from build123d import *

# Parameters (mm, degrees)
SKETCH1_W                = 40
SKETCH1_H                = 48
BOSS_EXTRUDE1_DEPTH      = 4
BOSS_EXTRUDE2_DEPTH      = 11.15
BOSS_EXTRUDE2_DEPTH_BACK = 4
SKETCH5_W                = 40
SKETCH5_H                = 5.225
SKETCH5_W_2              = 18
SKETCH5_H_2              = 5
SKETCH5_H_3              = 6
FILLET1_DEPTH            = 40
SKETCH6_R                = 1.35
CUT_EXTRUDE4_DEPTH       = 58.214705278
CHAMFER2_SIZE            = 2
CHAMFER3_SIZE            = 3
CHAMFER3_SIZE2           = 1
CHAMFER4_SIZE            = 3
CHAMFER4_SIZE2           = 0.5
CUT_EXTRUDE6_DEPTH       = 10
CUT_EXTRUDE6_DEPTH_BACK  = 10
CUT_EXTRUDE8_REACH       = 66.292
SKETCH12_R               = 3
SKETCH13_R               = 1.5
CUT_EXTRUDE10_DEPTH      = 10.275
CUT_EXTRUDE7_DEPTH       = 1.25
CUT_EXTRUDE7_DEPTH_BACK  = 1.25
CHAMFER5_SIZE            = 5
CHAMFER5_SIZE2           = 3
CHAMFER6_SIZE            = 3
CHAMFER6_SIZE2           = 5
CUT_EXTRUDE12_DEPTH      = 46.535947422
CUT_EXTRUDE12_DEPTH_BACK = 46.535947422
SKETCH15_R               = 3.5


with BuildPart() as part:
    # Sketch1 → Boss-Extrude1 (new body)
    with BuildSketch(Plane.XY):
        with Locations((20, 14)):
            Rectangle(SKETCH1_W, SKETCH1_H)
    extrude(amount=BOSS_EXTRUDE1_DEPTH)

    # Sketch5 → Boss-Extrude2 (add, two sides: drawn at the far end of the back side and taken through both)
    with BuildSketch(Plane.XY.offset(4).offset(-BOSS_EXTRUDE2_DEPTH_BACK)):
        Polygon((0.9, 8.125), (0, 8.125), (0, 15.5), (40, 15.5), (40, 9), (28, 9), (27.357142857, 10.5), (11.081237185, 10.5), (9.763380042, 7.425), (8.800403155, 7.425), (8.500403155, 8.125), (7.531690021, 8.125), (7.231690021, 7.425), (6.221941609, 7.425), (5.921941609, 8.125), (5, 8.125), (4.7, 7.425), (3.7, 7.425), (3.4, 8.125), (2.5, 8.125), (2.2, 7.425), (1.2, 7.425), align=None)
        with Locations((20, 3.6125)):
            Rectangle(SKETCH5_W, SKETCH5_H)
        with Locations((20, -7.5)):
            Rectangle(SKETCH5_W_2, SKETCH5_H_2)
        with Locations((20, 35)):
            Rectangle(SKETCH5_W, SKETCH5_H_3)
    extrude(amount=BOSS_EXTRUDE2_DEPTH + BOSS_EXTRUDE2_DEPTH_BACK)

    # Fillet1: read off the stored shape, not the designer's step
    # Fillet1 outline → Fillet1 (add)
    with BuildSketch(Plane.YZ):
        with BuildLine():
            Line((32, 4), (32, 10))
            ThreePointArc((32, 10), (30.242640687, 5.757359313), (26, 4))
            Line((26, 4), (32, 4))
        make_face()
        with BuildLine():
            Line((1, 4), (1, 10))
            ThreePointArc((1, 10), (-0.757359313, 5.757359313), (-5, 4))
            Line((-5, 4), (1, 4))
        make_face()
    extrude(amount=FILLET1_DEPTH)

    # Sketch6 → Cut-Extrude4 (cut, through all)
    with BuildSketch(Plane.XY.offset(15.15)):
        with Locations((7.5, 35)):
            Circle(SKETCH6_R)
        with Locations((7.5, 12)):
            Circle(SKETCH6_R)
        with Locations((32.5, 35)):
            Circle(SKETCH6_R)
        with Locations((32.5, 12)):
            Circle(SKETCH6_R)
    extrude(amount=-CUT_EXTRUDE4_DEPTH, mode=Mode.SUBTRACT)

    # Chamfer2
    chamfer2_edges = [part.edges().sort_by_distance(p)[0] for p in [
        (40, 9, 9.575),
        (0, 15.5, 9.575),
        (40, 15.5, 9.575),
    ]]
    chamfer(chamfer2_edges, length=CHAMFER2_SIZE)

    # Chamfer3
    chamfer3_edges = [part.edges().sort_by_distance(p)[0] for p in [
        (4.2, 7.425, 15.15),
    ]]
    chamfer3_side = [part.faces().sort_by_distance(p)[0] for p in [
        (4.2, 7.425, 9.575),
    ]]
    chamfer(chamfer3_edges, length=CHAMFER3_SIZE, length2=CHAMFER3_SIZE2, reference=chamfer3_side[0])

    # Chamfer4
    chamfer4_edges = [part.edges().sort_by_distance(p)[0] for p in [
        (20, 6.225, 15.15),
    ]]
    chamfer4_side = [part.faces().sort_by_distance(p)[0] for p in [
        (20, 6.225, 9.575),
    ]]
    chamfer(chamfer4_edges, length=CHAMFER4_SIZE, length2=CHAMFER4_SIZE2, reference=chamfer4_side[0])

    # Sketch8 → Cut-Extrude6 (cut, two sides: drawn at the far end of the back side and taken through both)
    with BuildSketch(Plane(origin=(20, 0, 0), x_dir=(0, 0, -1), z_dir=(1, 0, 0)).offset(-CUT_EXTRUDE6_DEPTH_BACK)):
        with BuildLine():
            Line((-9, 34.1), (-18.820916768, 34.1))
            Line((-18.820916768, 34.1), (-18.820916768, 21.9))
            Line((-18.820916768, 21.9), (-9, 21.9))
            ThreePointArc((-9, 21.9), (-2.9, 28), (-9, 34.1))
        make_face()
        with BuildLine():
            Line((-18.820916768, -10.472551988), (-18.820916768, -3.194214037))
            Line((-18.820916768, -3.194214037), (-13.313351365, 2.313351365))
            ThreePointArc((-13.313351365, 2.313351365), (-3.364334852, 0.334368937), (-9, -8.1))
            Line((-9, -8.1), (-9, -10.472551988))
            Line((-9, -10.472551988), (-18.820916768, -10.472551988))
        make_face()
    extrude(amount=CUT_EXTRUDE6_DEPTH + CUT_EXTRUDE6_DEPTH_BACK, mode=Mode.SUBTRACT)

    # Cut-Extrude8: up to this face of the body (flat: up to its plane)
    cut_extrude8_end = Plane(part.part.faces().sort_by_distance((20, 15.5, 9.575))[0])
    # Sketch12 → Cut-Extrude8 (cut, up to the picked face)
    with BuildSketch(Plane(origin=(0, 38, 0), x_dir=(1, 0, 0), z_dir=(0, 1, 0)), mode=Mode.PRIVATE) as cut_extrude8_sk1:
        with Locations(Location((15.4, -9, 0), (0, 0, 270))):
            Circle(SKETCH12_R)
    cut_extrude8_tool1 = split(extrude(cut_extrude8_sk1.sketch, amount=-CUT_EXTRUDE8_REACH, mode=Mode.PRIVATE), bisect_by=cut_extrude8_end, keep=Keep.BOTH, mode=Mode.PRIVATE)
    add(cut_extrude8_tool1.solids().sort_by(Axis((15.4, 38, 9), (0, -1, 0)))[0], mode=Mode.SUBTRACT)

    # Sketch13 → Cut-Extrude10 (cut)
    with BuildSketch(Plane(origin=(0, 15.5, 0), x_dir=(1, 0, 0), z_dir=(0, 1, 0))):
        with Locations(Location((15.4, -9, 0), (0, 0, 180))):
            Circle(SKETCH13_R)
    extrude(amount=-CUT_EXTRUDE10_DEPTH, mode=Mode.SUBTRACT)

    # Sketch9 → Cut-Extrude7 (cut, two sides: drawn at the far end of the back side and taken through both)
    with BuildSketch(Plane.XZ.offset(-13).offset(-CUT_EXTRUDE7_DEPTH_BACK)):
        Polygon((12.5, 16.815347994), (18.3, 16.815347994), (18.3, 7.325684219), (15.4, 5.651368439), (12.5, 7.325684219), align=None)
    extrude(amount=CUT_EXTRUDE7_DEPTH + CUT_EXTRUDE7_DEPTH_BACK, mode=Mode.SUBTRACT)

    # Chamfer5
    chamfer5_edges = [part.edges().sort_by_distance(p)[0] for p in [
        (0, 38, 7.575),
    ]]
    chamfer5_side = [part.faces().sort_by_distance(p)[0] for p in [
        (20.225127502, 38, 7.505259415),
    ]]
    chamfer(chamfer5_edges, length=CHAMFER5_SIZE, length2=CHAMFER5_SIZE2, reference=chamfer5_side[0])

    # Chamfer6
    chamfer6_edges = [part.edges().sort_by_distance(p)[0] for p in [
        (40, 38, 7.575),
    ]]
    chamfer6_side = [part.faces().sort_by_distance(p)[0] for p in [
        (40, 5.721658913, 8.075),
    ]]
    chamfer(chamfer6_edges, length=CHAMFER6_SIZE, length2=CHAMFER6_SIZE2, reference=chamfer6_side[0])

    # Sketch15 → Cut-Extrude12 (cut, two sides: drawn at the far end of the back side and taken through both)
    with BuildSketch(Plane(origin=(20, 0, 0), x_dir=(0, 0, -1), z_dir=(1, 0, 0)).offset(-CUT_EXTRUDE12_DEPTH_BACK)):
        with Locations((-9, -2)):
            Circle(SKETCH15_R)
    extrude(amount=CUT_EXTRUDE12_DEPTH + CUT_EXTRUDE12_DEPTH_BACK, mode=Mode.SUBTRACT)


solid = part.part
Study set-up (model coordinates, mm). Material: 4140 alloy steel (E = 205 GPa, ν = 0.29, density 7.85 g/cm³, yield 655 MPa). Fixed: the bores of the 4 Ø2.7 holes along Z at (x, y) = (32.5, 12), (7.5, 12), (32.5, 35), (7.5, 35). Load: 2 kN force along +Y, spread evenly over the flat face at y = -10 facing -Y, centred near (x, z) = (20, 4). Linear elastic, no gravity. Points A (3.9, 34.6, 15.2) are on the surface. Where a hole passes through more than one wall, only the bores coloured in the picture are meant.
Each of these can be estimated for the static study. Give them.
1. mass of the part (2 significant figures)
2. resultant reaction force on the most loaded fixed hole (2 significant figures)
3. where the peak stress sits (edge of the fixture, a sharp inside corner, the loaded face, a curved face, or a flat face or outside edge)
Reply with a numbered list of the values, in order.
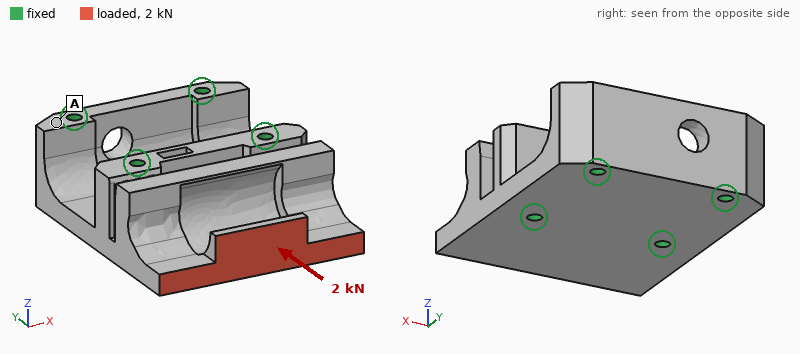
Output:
1. 110 g
2. 890 N
3. a curved face
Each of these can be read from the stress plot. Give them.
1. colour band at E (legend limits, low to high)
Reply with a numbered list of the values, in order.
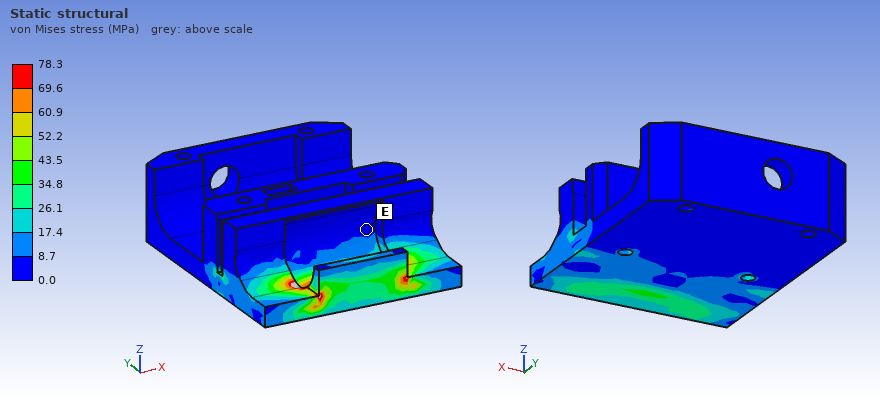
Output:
1. 0.0 to 8.7 MPa
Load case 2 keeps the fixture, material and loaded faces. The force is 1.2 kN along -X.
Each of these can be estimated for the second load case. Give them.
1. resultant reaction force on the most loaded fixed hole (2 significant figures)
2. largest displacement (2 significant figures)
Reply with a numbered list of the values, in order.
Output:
1. 1.0 kN
2. 7.2 µm
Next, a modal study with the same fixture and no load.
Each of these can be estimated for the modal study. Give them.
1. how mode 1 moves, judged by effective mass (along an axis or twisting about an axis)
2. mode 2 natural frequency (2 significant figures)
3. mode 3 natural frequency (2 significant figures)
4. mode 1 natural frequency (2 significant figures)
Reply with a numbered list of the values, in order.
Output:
1. along Z
2. 11 kHz
3. 21 kHz
4. 6100 Hz
